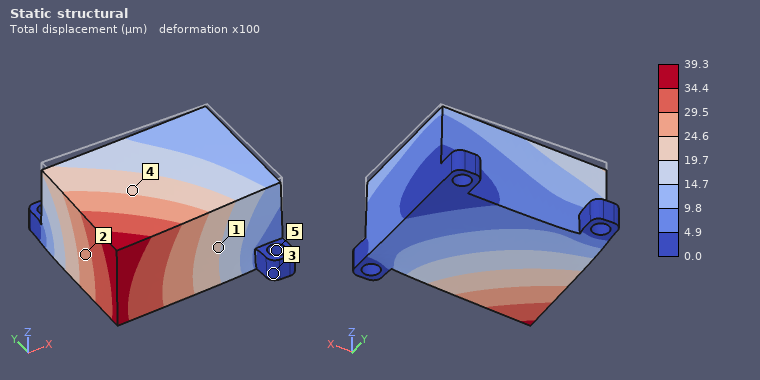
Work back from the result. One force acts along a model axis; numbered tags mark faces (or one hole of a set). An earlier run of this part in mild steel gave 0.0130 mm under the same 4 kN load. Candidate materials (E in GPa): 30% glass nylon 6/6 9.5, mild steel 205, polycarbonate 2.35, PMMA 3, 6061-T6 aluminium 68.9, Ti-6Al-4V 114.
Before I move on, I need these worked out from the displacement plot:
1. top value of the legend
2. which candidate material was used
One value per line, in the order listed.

39.3 µm
6061-T6 aluminium
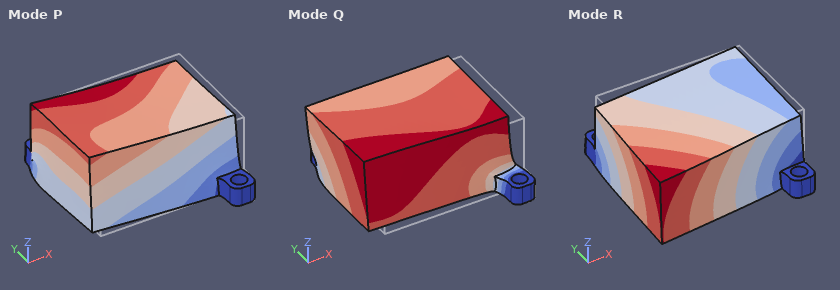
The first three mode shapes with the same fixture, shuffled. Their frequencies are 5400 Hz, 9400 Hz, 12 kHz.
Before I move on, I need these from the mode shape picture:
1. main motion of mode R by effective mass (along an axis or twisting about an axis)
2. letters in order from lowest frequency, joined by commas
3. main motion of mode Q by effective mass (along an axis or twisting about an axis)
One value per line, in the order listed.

along Z
R, Q, P
along X
